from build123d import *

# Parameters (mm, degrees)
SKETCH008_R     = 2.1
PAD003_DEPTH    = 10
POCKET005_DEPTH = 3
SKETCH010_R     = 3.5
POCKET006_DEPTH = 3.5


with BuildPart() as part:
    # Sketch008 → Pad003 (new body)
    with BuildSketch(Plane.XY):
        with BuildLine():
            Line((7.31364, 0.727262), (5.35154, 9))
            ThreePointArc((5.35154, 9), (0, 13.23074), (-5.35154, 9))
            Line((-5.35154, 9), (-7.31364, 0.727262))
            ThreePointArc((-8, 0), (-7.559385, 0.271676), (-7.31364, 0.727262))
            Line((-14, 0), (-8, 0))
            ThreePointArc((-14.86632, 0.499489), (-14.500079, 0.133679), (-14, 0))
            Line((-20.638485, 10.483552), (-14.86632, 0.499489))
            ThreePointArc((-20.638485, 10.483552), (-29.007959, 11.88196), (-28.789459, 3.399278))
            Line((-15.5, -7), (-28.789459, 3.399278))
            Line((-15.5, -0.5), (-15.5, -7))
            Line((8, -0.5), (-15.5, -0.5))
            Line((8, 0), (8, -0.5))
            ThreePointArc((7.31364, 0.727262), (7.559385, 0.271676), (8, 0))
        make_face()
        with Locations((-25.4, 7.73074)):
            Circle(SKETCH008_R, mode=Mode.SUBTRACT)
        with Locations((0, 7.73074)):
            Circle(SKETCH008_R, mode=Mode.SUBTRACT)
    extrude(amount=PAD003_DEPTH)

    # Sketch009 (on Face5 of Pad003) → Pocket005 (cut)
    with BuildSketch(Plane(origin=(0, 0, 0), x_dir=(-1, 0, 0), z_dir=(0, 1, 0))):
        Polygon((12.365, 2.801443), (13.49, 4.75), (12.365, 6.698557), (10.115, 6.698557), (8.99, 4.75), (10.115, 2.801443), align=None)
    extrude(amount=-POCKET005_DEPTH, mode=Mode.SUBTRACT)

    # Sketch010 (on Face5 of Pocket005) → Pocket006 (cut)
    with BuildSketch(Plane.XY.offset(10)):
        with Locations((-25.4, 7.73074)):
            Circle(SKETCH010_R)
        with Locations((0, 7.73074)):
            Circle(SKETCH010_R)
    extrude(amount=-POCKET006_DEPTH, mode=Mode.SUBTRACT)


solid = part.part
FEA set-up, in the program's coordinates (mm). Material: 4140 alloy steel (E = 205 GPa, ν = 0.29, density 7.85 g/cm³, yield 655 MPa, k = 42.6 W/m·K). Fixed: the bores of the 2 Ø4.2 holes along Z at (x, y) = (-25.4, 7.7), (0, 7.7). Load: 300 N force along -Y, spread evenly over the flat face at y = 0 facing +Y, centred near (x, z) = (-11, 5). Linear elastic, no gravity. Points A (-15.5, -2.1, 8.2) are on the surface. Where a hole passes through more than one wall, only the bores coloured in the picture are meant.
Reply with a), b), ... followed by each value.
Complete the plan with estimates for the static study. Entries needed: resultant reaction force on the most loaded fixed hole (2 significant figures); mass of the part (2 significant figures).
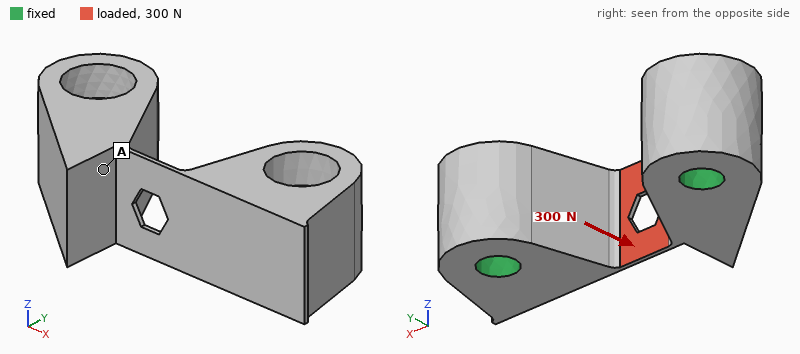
a) 200 N
b) 23 g
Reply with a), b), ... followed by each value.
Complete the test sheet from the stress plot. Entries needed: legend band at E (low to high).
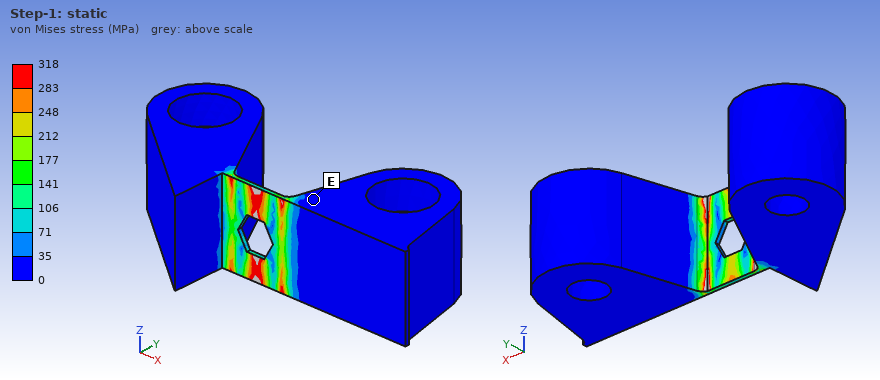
a) 0 to 35 MPa
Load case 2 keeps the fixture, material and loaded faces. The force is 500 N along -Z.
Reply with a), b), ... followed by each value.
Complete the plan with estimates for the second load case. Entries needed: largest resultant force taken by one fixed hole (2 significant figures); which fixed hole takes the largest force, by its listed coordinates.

a) 280 N
b) (0, 7.7)
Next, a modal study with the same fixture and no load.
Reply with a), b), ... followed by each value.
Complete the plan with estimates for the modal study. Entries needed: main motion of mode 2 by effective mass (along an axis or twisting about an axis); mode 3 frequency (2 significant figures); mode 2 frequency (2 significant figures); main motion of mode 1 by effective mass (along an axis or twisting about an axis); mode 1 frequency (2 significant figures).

a) along X
b) 45 kHz
c) 28 kHz
d) along Z
e) 27 kHz
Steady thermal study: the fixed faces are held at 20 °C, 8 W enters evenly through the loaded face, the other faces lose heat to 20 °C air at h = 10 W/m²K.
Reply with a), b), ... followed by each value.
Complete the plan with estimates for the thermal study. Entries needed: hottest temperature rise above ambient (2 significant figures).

a) 71 K
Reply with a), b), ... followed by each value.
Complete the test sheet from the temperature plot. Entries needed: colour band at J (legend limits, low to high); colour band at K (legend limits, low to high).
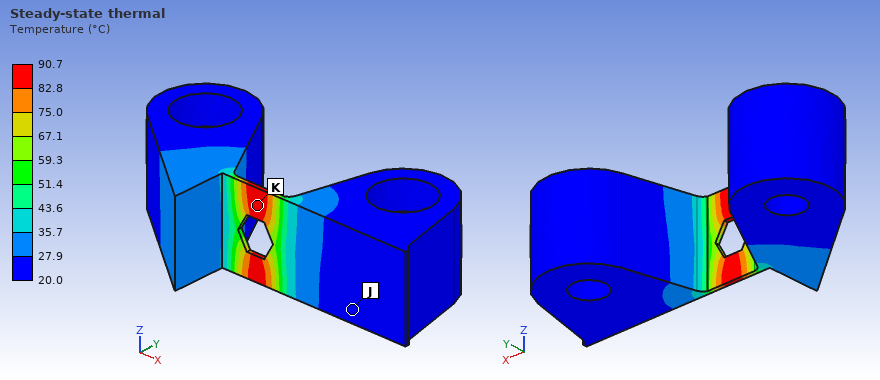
a) 20.0 to 27.9 °C
b) 82.8 to 90.7 °C
